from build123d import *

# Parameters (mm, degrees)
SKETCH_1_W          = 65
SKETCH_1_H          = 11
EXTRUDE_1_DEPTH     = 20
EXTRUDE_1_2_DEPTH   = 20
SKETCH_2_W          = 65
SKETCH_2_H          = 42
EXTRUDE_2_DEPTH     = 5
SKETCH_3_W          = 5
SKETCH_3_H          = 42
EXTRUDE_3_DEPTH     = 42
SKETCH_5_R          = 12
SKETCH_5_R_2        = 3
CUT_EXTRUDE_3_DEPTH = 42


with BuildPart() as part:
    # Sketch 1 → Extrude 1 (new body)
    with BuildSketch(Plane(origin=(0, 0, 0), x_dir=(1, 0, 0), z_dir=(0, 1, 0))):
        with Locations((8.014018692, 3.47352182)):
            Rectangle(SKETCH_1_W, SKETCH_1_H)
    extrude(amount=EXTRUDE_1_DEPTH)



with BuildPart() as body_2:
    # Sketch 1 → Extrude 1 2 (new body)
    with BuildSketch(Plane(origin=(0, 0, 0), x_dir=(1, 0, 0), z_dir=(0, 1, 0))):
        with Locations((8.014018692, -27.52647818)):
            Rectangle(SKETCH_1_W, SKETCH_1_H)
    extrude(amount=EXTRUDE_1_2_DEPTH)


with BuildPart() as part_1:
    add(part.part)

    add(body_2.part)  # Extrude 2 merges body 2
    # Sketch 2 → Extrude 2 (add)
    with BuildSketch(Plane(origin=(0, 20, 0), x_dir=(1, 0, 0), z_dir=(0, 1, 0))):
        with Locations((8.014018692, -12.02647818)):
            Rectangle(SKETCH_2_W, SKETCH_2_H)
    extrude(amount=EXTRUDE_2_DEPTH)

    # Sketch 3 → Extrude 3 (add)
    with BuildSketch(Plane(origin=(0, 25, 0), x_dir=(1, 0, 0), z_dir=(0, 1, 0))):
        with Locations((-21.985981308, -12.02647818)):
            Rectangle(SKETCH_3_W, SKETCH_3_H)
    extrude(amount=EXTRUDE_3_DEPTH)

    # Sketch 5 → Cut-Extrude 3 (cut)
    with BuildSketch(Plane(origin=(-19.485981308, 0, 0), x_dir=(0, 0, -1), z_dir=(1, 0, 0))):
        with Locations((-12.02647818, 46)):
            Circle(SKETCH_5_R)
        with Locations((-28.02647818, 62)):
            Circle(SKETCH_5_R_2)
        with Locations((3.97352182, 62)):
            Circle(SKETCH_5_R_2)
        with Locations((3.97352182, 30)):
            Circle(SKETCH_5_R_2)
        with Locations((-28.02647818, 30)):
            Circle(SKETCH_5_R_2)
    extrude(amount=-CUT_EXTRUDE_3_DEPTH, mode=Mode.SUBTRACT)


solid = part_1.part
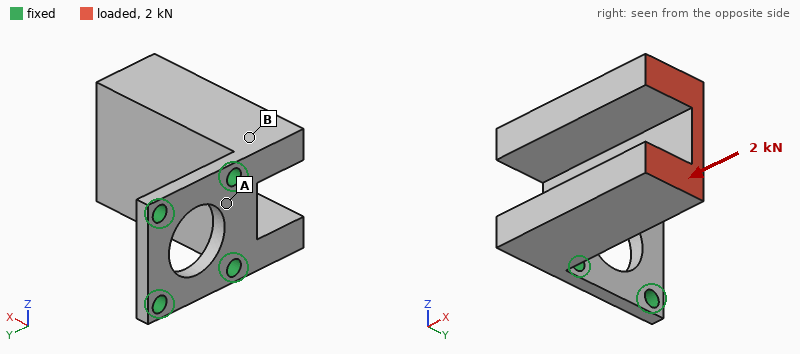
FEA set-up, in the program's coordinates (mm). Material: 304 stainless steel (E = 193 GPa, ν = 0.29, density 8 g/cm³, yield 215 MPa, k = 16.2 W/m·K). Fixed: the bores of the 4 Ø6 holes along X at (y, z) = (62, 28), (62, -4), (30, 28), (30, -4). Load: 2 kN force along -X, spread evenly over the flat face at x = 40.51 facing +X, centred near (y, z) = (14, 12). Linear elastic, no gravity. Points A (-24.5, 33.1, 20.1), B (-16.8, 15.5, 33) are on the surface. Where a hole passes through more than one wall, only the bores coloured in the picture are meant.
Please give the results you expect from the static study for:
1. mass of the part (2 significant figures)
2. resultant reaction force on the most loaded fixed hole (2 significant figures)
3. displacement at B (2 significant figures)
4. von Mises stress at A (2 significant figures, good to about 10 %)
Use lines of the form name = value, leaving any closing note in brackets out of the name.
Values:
mass of the part = 390 g
resultant reaction force on the most loaded fixed hole = 1.0 kN
displacement at B = 0.026 mm
von Mises stress at A = 41 MPa
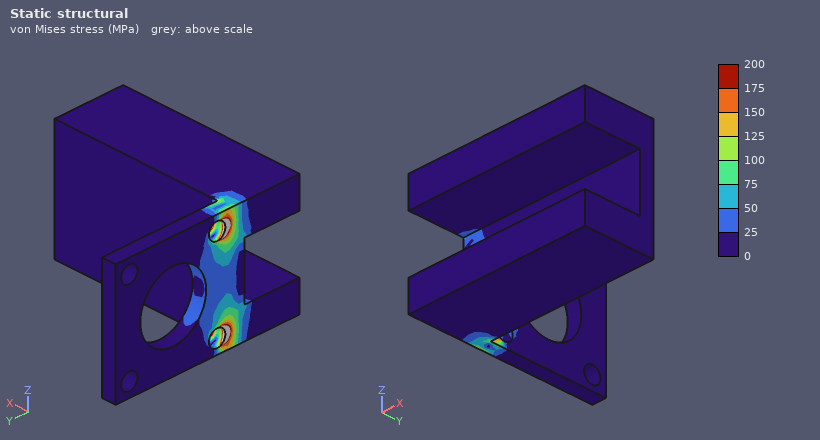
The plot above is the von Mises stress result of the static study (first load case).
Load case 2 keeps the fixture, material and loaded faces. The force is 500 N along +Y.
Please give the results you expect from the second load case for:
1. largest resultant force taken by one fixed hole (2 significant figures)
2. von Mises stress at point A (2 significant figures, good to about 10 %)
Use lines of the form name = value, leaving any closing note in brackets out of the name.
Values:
largest resultant force taken by one fixed hole = 260 N
von Mises stress at point A = 45 MPa
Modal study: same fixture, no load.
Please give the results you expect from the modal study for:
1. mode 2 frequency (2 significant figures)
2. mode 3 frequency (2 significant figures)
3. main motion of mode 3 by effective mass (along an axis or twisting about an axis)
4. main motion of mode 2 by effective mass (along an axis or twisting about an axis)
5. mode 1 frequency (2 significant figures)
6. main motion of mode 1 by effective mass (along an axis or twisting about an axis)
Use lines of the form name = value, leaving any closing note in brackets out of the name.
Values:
mode 2 frequency = 2600 Hz
mode 3 frequency = 2900 Hz
main motion of mode 3 by effective mass = along Z
main motion of mode 2 by effective mass = along Z
mode 1 frequency = 740 Hz
main motion of mode 1 by effective mass = along Y
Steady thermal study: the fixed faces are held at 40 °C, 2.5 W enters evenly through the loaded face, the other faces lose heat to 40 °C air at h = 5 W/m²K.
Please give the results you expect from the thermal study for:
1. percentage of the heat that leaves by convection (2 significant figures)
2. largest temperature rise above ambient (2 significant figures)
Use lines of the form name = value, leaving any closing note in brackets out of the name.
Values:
percentage of the heat that leaves by convection = 26 %
largest temperature rise above ambient = 18 K
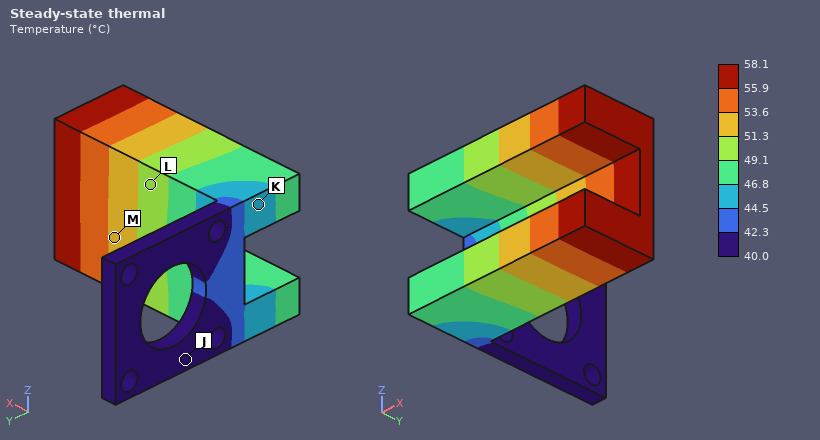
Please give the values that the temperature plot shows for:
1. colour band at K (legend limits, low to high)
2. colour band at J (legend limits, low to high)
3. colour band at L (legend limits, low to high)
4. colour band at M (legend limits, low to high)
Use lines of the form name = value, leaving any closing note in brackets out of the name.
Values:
colour band at K = 44.5 to 46.8 °C
colour band at J = 40.0 to 42.3 °C
colour band at L = 49.1 to 51.3 °C
colour band at M = 51.3 to 53.6 °C
